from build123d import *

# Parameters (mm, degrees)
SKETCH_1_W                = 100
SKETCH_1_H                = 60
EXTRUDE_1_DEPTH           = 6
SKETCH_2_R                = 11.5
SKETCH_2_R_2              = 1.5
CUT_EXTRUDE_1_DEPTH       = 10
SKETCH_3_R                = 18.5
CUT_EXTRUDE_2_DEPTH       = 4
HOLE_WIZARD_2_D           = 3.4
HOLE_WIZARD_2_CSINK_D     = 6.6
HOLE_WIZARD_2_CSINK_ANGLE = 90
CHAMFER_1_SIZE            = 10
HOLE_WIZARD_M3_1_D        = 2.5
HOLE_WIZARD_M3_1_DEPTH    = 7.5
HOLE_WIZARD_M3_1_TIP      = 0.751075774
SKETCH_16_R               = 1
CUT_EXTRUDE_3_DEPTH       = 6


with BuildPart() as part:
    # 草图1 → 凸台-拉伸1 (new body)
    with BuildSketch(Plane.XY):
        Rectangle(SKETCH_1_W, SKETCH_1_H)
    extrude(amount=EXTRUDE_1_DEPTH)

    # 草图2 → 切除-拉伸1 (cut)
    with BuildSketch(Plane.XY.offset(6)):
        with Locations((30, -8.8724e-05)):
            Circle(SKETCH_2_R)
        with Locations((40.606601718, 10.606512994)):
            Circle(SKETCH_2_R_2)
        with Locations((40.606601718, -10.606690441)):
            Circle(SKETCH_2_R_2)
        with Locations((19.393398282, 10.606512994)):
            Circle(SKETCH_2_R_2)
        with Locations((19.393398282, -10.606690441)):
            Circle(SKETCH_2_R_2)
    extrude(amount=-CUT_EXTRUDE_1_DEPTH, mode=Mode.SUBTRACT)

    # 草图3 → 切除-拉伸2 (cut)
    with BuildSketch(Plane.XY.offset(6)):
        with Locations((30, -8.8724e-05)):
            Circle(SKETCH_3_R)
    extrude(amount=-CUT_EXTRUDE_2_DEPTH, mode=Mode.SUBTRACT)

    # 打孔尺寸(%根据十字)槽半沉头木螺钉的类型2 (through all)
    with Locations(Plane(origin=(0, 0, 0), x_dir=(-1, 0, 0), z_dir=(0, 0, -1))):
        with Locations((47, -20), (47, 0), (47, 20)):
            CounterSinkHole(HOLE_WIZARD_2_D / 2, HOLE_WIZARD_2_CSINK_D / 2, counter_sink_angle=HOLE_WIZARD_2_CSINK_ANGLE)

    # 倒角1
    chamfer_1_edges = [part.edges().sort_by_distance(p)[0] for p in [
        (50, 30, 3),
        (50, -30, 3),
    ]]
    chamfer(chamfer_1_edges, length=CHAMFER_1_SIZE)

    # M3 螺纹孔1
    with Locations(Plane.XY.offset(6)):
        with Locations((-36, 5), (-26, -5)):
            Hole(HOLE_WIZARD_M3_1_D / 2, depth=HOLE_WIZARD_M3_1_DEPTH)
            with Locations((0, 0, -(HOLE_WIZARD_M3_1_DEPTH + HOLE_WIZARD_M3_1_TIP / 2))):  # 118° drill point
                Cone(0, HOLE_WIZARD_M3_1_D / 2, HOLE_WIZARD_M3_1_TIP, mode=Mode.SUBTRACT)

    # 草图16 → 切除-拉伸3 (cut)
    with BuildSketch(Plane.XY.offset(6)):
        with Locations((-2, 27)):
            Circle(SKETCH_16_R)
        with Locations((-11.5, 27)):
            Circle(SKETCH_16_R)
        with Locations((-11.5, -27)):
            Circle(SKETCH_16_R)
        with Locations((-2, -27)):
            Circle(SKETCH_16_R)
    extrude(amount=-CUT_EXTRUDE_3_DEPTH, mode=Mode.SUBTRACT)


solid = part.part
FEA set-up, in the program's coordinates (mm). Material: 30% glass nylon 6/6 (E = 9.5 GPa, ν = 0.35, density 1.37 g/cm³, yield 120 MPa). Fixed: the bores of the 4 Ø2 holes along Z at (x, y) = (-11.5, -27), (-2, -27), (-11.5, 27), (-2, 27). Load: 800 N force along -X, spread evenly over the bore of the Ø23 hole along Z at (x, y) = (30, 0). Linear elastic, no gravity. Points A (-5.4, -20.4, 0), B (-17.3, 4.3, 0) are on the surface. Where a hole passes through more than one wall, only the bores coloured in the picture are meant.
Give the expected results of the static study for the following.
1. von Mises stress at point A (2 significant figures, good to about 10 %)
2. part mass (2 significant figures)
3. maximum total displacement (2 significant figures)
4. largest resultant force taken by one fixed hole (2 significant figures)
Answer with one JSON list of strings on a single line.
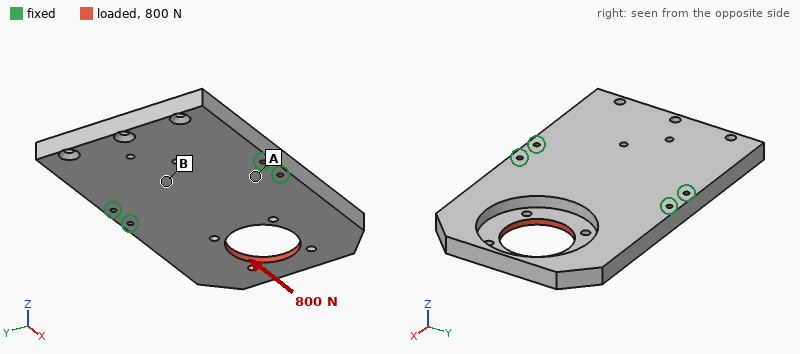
["5.1 MPa", "41 g", "0.25 mm", "260 N"]
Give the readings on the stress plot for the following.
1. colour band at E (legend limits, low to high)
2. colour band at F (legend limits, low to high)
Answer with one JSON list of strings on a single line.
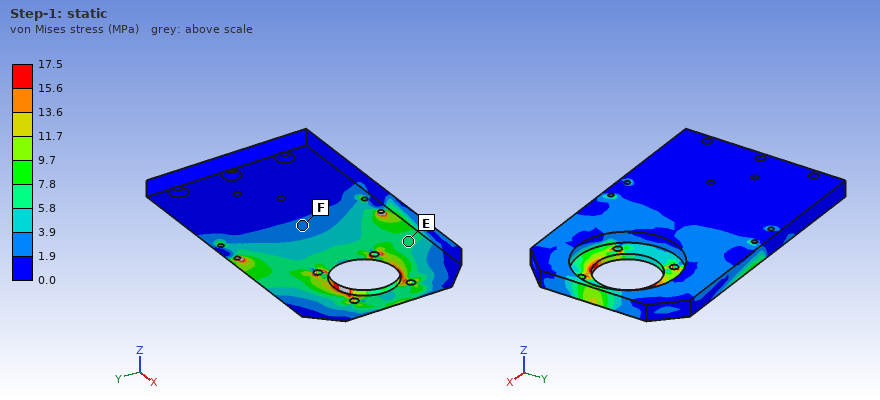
["5.8 to 7.8 MPa", "1.9 to 3.9 MPa"]
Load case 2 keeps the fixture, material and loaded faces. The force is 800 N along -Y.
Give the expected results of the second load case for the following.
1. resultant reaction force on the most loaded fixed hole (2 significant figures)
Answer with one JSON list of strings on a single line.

["500 N"]
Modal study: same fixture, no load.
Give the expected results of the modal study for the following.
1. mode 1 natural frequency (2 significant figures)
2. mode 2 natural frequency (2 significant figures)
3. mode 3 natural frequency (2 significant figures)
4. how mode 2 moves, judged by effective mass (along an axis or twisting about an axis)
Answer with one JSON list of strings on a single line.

["900 Hz", "1300 Hz", "1800 Hz", "along Z"]
